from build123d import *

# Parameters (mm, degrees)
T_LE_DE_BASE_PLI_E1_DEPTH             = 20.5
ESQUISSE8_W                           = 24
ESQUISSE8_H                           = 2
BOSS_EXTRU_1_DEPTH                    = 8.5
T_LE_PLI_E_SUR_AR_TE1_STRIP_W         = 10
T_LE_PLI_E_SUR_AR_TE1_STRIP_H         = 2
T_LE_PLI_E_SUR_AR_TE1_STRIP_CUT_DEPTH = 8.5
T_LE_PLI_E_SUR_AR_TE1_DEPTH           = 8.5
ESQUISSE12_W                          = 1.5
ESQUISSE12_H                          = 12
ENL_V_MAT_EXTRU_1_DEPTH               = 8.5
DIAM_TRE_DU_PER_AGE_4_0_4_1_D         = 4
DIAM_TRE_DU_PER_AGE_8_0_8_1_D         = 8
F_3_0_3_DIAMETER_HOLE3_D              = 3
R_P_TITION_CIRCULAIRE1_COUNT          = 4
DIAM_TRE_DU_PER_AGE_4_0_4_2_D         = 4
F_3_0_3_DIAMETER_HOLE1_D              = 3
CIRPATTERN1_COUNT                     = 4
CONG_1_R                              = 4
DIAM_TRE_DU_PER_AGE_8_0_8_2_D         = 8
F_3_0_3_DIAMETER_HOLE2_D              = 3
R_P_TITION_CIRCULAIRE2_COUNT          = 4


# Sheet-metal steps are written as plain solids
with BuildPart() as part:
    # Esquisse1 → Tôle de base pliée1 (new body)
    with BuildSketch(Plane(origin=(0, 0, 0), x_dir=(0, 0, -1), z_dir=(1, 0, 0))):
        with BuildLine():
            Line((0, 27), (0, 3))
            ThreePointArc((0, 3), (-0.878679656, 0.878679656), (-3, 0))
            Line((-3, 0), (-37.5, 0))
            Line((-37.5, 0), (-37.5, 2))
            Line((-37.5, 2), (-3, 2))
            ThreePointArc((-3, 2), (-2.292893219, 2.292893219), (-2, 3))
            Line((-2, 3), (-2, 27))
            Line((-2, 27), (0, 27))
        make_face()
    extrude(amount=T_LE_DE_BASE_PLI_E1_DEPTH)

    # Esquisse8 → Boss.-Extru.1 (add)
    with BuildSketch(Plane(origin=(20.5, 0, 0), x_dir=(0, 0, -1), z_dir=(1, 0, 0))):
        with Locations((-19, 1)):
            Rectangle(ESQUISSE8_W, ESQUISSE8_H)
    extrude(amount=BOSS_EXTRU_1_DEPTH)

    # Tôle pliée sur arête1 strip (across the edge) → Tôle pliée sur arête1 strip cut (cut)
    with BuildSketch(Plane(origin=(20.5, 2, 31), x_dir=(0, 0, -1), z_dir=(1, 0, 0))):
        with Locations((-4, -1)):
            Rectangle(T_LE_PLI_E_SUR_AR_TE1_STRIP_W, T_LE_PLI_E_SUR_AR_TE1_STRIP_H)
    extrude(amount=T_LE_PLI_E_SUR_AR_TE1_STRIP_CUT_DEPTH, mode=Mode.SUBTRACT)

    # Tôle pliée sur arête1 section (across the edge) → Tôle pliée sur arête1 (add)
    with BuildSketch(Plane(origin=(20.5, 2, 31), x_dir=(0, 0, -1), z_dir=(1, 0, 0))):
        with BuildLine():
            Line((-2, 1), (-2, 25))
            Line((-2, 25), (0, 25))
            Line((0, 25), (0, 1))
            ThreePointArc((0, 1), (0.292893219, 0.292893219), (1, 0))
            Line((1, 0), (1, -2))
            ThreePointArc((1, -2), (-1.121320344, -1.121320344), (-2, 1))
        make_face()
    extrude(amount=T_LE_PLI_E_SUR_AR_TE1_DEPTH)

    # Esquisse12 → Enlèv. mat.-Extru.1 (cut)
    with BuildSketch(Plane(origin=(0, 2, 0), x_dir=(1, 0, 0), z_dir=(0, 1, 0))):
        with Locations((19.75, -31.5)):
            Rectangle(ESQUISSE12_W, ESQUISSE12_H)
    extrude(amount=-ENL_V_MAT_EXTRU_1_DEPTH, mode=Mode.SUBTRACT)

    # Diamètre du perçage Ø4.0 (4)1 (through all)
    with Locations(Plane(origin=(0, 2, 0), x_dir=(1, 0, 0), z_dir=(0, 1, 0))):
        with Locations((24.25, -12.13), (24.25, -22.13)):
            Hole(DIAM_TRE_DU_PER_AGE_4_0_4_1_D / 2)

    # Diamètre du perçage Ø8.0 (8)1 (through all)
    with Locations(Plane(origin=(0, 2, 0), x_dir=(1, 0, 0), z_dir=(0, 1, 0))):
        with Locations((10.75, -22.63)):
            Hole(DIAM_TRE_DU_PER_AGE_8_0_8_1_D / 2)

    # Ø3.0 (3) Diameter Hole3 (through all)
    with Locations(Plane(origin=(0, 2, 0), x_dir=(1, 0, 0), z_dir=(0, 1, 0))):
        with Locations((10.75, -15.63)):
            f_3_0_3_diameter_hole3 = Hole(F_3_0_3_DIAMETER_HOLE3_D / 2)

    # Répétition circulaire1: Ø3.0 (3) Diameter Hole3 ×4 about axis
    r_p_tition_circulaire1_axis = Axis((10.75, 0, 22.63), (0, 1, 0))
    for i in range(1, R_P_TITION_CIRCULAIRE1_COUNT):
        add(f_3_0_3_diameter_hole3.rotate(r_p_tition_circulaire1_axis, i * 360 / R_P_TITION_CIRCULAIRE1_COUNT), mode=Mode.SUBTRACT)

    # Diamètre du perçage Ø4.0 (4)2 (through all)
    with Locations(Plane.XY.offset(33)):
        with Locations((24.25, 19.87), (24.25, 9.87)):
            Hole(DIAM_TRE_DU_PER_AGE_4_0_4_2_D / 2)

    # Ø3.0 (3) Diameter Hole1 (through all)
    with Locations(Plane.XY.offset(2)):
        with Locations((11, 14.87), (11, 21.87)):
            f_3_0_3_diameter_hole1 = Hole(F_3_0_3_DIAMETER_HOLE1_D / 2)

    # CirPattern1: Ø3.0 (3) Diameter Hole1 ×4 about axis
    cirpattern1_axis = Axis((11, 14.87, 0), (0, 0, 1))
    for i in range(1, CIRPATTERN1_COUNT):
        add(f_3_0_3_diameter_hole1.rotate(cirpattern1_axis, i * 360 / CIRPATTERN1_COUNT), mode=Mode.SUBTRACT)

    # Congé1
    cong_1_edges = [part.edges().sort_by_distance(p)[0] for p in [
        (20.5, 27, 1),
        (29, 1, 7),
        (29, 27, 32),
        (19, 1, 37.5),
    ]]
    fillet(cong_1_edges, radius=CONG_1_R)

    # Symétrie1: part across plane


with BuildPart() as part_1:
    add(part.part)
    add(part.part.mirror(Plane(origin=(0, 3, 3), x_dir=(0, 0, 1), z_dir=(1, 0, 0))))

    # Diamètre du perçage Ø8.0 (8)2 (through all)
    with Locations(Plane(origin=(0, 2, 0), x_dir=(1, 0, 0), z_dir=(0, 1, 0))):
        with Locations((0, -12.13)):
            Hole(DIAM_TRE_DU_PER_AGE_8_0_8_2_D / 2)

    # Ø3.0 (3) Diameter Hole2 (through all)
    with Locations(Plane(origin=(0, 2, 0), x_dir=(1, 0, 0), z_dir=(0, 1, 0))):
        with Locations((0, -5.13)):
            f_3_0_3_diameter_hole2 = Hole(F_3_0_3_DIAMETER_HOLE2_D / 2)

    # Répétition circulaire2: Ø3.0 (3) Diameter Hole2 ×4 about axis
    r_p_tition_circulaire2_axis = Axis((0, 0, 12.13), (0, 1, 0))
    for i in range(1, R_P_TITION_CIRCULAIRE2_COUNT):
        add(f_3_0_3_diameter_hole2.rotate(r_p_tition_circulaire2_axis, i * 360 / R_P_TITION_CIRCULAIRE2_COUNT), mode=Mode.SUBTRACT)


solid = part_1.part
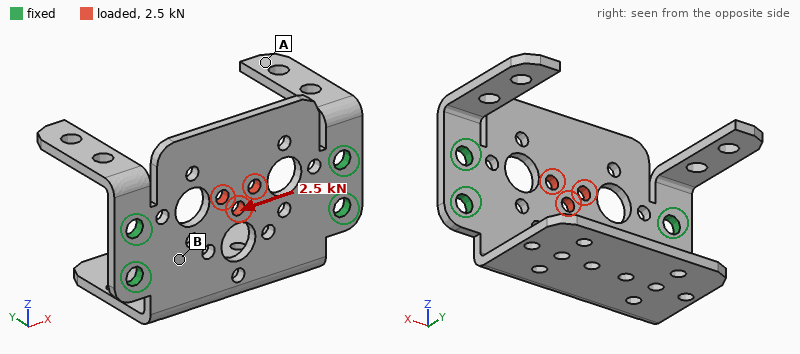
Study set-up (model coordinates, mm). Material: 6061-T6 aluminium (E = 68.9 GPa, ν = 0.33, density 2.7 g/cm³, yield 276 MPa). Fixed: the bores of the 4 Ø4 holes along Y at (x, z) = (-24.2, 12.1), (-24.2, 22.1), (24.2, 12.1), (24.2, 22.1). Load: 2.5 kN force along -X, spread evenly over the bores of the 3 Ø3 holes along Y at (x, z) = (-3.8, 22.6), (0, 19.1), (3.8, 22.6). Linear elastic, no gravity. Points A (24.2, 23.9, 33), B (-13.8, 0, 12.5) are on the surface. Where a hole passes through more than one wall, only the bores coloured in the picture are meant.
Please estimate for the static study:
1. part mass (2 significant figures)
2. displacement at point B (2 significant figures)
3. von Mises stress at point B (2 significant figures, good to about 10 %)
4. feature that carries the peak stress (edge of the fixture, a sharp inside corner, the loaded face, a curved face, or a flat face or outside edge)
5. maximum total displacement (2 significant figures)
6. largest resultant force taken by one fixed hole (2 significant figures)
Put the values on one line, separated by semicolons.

16 g; 5.8 µm; 39 MPa; a curved face; 31 µm; 680 N
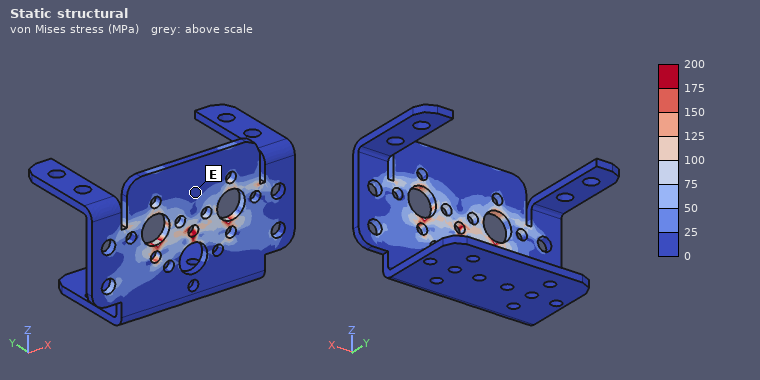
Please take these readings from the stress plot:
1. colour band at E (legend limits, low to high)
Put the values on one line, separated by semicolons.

0 to 25 MPa
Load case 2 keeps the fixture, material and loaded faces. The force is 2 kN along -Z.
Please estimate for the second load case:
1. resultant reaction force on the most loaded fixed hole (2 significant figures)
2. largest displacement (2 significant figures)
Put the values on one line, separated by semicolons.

560 N; 37 µm
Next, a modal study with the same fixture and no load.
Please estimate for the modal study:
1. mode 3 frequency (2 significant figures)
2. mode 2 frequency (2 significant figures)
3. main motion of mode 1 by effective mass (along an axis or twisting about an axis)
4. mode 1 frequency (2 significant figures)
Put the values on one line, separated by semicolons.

1700 Hz; 1700 Hz; along Z; 1300 Hz
